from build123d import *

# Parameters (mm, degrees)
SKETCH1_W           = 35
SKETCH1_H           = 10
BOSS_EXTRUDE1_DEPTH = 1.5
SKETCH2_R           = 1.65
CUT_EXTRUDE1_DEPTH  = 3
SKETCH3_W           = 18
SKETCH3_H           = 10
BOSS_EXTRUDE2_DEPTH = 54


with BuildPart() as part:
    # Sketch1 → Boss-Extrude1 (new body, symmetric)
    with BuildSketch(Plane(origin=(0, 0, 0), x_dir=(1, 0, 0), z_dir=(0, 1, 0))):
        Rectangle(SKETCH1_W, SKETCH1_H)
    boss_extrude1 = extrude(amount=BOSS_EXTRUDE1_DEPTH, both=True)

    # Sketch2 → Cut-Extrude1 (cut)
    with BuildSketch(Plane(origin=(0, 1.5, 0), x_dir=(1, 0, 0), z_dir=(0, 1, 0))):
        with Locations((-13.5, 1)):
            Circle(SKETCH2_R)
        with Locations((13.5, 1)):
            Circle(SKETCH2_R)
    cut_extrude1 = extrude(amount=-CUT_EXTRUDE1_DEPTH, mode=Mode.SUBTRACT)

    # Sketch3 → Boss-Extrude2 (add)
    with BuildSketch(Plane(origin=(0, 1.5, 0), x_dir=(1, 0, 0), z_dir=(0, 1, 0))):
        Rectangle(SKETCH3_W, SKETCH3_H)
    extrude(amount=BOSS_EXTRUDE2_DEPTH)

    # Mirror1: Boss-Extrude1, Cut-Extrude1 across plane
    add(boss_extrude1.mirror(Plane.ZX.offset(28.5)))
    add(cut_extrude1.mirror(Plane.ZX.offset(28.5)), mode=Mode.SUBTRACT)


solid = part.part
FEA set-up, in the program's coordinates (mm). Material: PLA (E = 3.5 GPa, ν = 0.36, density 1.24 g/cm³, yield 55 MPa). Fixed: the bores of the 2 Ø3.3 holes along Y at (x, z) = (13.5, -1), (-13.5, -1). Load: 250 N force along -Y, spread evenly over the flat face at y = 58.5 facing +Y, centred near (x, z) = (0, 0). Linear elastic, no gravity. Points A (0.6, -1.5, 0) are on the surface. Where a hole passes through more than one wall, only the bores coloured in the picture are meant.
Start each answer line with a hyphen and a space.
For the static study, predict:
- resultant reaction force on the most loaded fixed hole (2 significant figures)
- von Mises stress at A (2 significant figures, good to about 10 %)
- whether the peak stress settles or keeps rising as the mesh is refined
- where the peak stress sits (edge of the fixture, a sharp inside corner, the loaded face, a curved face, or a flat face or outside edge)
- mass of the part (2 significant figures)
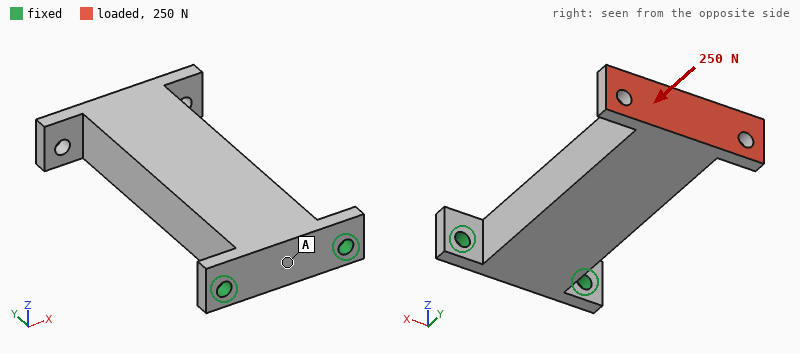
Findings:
- 140 N
- 2.2 MPa
- keeps rising
- edge of the fixture
- 15 g
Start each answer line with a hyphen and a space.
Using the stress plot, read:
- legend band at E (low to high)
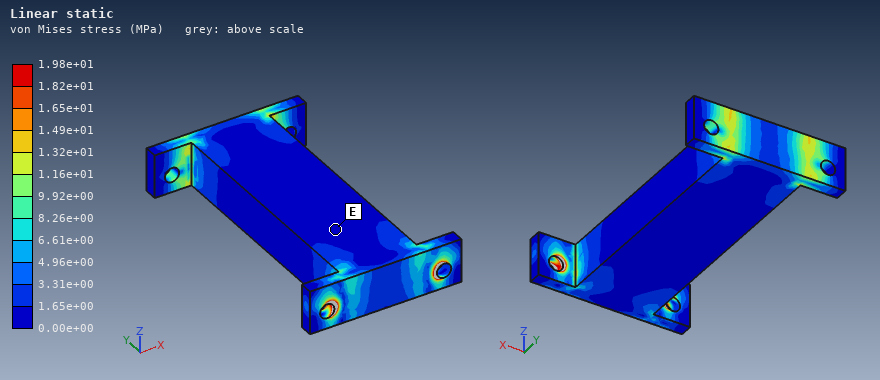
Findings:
- 0.00e+00 to 1.65e+00 MPa
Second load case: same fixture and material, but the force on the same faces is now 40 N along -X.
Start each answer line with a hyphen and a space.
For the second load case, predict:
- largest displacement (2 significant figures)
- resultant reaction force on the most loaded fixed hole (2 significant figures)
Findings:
- 0.38 mm
- 110 N
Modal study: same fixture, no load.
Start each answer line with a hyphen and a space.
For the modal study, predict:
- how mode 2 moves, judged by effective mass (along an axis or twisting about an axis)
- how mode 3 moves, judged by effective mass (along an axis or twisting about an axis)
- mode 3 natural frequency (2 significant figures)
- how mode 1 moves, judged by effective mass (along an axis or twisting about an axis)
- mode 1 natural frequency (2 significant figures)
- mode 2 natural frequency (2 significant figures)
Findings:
- along X
- twisting about Y
- 2700 Hz
- along Z
- 270 Hz
- 800 Hz
